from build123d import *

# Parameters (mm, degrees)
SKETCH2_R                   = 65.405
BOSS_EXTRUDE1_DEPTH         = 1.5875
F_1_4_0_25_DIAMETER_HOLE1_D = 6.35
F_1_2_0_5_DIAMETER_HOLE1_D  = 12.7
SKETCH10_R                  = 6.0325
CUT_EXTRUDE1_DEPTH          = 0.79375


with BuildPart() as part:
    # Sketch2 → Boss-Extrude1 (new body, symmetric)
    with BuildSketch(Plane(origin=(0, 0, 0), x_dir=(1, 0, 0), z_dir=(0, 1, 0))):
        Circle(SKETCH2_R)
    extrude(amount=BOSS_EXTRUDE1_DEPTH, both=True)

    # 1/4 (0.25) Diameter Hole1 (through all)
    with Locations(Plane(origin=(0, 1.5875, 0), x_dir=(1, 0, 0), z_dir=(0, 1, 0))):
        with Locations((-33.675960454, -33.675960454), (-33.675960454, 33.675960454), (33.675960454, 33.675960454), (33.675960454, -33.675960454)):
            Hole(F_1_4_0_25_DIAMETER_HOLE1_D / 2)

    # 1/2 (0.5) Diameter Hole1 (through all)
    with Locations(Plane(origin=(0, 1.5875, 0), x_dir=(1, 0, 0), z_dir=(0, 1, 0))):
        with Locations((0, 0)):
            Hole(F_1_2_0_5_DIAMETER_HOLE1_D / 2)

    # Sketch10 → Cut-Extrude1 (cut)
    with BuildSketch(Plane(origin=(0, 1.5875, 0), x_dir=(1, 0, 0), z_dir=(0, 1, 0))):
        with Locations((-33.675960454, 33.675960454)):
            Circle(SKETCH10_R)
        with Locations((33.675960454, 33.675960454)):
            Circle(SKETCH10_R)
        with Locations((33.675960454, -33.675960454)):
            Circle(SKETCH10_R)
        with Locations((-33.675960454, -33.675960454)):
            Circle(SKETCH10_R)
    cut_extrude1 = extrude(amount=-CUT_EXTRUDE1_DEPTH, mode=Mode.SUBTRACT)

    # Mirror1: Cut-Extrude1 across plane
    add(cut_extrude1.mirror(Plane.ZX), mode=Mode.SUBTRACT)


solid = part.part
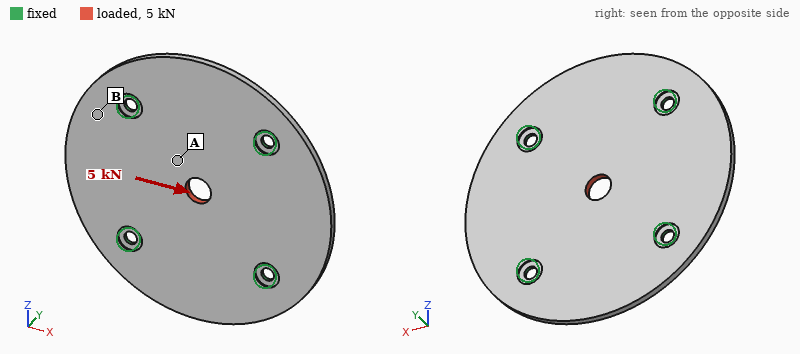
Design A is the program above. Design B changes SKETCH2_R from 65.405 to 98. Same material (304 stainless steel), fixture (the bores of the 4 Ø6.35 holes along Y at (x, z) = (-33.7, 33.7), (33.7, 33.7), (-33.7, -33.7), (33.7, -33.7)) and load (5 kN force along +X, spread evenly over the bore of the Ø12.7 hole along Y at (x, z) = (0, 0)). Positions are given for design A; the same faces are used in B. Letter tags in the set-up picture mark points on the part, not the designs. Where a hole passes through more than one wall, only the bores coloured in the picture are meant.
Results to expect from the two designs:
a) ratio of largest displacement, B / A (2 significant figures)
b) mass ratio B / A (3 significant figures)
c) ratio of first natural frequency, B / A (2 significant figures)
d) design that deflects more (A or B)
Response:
10
2.29
0.35
B
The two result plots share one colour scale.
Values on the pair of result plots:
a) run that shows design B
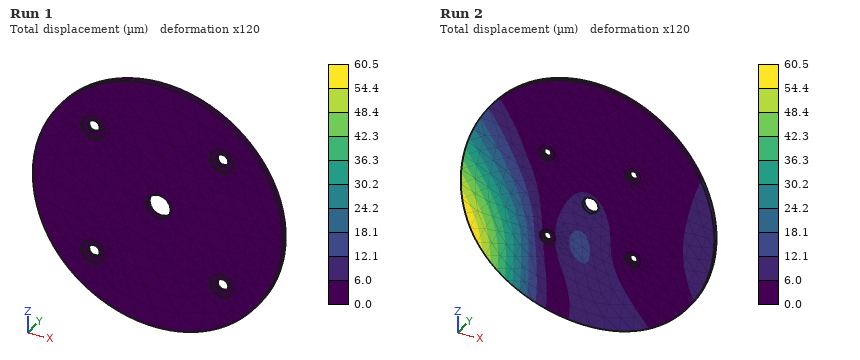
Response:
Run 2
